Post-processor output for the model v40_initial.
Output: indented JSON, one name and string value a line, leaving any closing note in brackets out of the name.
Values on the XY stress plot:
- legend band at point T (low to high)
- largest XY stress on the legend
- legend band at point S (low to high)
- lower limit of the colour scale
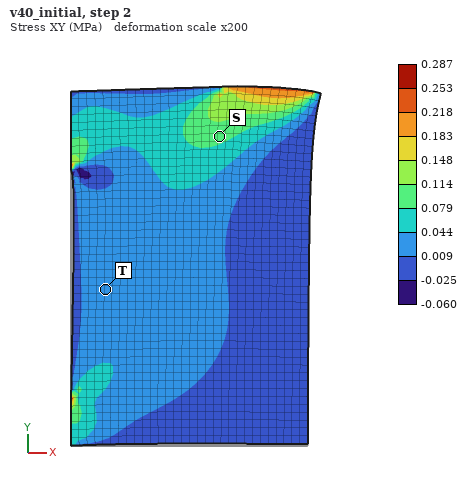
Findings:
{
  "legend band at point T": "0.009 to 0.044 MPa",
  "largest XY stress on the legend": "0.287 MPa",
  "legend band at point S": "0.079 to 0.114 MPa",
  "lower limit of the colour scale": "-0.060 MPa"
}
